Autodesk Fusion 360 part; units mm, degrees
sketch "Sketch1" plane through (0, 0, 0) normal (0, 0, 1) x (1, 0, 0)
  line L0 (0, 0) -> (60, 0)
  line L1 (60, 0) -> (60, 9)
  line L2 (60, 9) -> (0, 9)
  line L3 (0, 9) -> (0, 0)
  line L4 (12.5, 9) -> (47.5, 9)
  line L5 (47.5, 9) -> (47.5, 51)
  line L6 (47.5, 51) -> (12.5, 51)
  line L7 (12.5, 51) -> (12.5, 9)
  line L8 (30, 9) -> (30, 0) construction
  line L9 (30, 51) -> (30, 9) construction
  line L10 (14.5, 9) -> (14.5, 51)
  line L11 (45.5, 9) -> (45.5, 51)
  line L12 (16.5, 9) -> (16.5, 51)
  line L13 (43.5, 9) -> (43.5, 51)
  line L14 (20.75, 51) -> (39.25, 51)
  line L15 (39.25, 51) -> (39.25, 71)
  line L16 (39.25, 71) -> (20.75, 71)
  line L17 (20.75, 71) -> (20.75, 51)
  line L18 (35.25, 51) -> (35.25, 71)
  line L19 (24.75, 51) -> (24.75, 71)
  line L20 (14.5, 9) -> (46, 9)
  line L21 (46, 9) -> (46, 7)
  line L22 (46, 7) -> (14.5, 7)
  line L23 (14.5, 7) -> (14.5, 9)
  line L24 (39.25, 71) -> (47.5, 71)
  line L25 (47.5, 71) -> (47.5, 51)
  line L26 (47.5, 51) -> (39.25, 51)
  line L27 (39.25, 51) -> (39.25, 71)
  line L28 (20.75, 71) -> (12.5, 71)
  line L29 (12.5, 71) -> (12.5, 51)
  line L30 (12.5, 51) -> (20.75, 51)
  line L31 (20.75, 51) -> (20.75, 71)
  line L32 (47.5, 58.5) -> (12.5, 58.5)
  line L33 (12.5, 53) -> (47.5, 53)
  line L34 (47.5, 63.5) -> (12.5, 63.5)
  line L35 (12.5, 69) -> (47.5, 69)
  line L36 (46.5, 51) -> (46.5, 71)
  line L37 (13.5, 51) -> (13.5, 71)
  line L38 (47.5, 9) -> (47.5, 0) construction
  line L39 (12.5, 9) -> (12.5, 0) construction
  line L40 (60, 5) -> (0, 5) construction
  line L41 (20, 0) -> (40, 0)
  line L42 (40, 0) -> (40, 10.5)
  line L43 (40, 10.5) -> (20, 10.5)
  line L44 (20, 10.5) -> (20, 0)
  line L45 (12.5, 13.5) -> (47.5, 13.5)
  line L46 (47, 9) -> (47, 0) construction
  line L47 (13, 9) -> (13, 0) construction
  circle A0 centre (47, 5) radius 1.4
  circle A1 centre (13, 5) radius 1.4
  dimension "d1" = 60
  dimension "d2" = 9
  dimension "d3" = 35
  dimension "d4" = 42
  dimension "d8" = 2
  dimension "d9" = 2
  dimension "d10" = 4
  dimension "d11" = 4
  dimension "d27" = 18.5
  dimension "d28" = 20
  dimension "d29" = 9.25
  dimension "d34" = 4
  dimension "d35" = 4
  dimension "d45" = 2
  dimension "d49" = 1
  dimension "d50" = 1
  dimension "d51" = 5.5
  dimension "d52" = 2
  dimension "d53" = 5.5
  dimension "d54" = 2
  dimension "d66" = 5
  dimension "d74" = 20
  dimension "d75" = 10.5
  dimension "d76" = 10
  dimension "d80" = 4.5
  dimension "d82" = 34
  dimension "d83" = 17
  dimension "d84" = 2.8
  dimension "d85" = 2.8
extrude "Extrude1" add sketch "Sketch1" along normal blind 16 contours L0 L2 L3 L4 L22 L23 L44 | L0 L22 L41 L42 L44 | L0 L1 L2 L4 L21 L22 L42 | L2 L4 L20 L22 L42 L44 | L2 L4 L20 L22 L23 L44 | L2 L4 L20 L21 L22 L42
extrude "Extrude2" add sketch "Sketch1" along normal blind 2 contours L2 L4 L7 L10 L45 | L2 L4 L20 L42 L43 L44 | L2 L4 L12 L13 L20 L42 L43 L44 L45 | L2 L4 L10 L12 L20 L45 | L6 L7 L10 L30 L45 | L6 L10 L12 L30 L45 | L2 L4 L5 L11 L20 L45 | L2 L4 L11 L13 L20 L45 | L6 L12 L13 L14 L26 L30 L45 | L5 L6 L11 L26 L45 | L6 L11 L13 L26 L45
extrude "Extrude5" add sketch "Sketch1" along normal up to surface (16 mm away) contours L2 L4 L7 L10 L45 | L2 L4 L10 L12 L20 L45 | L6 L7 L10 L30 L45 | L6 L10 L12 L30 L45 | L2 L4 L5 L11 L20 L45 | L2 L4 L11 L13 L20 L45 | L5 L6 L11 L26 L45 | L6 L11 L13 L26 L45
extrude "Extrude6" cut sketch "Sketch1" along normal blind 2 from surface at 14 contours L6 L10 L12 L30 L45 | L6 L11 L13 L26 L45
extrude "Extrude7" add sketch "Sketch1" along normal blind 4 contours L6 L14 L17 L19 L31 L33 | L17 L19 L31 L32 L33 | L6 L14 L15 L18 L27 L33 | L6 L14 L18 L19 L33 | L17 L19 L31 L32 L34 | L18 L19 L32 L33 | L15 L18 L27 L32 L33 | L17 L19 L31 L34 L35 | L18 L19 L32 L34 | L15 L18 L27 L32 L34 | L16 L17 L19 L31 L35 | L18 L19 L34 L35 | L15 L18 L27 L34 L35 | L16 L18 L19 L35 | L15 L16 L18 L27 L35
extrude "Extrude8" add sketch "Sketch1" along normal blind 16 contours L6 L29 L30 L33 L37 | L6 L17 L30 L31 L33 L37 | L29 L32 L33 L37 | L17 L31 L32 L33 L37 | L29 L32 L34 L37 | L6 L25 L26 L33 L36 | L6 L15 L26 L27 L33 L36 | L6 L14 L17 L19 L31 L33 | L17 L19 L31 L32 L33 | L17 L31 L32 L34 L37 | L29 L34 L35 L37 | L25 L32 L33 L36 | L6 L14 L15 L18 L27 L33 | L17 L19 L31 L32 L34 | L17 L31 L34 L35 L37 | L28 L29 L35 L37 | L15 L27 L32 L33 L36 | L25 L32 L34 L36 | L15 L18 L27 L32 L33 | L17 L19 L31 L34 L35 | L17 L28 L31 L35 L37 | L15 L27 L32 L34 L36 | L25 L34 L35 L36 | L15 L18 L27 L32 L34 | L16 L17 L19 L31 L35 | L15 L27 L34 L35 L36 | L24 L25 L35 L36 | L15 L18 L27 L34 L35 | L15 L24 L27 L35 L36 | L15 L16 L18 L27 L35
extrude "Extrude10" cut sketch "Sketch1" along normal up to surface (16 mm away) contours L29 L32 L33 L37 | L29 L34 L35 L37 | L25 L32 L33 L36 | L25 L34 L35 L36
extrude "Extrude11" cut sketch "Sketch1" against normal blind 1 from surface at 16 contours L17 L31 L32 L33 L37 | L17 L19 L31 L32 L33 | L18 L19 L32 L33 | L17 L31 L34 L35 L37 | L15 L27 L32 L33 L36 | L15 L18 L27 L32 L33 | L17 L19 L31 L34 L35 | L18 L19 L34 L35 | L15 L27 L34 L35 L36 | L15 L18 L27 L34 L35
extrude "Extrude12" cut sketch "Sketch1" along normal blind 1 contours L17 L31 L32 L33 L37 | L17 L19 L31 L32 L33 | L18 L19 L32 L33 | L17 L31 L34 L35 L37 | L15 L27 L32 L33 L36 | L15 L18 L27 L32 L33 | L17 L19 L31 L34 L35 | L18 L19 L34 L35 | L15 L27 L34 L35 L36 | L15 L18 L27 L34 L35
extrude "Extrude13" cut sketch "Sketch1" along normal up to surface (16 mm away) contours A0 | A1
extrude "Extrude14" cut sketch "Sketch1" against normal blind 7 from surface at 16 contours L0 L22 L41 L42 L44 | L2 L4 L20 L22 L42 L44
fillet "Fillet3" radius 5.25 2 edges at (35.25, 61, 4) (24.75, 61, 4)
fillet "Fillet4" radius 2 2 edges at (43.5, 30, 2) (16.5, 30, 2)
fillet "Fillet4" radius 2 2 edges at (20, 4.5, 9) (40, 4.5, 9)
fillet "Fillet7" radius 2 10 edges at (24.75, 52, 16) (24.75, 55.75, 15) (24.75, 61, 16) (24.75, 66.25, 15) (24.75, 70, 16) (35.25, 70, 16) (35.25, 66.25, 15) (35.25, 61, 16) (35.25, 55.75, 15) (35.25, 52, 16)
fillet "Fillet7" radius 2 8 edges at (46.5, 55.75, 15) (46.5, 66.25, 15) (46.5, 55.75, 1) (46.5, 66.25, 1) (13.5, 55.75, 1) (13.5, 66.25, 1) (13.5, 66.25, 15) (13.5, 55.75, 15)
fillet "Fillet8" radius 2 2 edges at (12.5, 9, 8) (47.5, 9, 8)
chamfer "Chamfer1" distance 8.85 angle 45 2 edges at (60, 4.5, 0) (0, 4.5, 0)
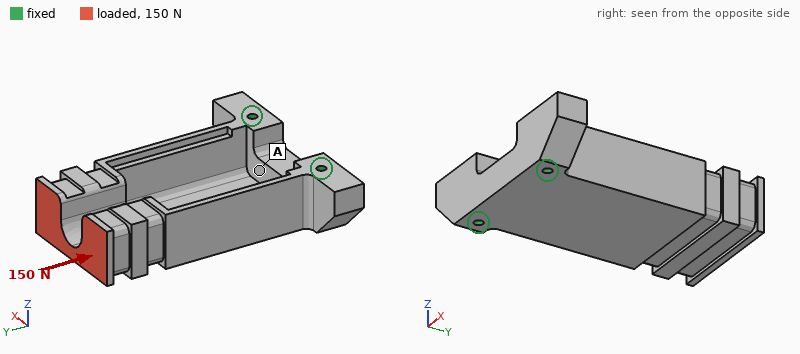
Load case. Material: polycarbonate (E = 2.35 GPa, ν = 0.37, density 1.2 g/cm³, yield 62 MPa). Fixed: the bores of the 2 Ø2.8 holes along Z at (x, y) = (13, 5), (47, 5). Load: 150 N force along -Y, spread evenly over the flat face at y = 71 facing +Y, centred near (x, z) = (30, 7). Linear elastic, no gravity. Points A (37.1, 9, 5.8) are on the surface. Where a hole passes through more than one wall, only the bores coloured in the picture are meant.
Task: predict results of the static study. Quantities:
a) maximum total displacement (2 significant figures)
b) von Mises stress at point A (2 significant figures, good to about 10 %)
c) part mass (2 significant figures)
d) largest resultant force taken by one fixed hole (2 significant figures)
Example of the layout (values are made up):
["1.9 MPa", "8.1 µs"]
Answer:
["65 µm", "0.24 MPa", "26 g", "75 N"]
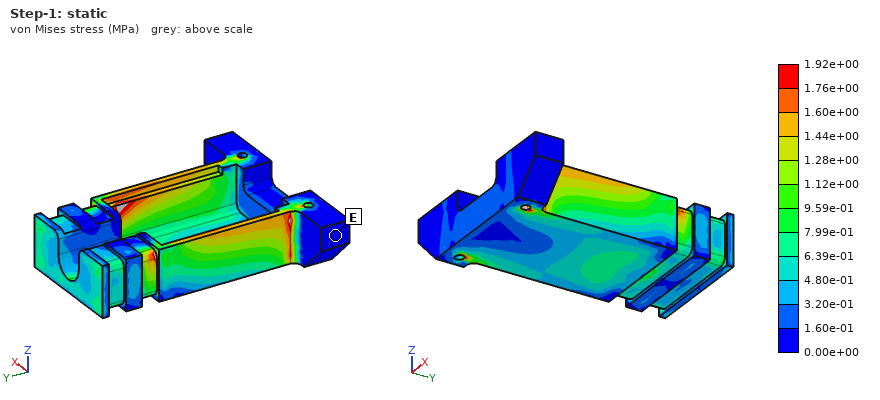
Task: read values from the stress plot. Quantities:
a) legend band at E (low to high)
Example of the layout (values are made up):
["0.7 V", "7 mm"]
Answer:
["0.00e+00 to 1.60e-01 MPa"]
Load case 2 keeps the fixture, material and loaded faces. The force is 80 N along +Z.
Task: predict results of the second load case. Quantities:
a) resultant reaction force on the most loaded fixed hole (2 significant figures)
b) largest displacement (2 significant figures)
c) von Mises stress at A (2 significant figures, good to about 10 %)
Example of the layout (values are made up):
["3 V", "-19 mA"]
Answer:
["54 N", "0.95 mm", "1.8 MPa"]
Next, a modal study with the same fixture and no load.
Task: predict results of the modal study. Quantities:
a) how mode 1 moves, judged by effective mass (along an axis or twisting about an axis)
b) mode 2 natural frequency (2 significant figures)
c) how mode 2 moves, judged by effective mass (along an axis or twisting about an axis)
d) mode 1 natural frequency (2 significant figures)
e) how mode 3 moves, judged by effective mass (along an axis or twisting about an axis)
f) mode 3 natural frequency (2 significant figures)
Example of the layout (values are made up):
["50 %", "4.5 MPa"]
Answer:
["along Z", "710 Hz", "along X", "560 Hz", "along X", "1700 Hz"]
